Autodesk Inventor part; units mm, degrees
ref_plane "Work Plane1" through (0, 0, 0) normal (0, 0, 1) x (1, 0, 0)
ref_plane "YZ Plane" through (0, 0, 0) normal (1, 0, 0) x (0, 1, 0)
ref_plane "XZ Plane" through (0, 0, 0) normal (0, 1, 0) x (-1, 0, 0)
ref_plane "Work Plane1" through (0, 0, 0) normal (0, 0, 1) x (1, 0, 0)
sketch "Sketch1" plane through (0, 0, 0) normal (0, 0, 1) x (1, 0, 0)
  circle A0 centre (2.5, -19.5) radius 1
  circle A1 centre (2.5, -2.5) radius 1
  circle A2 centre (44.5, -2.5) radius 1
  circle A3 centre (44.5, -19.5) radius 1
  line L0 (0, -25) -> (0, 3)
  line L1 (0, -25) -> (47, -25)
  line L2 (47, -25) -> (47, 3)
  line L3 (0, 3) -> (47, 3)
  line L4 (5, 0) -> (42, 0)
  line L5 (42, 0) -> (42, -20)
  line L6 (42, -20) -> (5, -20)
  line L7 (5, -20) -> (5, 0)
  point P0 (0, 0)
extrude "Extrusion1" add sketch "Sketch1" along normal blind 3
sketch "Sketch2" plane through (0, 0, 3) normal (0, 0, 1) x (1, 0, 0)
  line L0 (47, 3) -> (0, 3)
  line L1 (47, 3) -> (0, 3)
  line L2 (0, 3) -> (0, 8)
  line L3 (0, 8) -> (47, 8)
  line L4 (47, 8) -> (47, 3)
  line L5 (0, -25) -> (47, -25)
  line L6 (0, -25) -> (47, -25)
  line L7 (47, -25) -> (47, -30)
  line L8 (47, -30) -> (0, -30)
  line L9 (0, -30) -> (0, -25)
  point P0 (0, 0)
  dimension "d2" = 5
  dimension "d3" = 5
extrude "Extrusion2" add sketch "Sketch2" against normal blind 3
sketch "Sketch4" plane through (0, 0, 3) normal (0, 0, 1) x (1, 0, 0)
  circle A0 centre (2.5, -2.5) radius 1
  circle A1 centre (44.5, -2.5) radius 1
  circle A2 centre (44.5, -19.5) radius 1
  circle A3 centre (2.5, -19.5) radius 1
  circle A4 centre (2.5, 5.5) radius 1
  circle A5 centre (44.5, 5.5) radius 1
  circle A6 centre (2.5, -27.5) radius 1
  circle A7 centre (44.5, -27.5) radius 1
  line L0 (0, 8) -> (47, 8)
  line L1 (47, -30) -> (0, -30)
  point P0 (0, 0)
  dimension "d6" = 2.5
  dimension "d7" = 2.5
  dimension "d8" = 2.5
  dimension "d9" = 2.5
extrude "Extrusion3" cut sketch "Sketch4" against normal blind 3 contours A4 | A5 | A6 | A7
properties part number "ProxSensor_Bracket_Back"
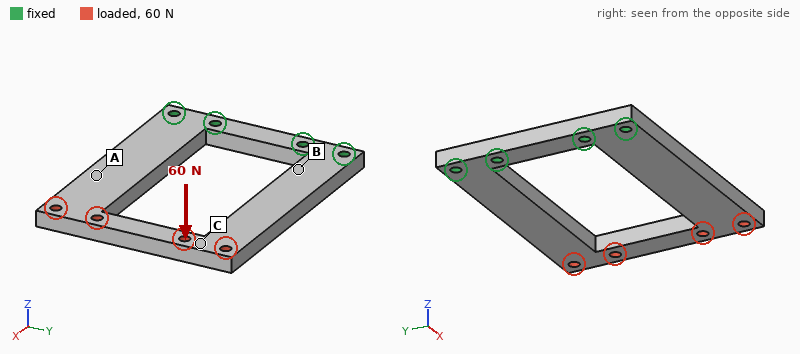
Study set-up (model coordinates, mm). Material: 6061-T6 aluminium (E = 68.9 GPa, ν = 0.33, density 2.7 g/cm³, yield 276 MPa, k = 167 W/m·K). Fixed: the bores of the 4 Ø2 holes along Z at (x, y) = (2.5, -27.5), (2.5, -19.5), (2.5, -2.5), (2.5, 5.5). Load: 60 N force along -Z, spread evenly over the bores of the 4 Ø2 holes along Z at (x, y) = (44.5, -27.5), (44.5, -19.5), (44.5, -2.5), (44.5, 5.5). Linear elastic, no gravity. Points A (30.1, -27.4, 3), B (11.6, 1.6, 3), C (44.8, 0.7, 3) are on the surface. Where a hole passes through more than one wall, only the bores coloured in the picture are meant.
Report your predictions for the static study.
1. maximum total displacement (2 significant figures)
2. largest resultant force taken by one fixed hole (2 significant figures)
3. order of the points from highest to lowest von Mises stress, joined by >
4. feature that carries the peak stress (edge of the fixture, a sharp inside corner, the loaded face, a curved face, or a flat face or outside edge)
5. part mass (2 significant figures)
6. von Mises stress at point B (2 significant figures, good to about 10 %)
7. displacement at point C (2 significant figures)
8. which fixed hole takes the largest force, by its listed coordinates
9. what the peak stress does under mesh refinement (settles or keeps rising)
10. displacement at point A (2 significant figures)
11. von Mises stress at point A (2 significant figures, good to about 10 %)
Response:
0.58 mm
35 N
B > A > C
edge of the fixture
8.3 g
74 MPa
0.54 mm
(2.5, 5.5)
keeps rising
0.26 mm
32 MPa
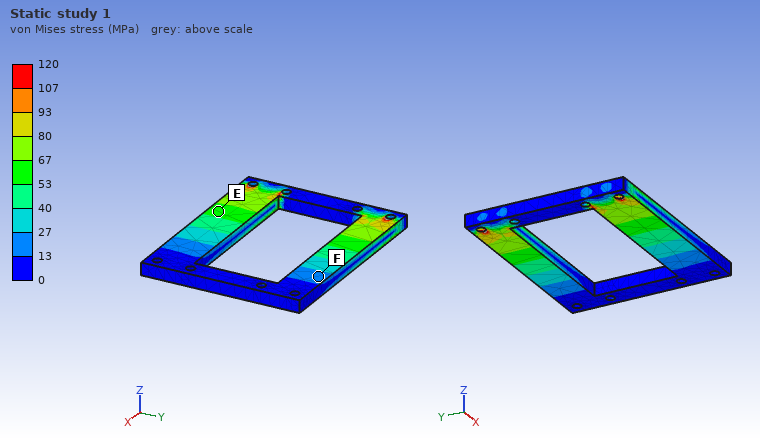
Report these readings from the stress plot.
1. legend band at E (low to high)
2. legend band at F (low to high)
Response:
53 to 67 MPa
13 to 27 MPa
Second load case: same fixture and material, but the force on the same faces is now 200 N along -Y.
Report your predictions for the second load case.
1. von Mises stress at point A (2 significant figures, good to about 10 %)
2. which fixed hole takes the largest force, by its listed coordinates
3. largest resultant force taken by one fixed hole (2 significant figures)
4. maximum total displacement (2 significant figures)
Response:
10.0 MPa
(2.5, -27.5)
480 N
0.11 mm
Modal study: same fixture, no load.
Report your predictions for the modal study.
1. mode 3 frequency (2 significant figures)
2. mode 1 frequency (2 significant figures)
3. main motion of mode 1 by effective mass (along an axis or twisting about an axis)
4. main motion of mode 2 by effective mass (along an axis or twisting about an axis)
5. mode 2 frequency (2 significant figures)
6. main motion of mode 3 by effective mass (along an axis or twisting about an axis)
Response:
4100 Hz
1100 Hz
along Z
twisting about X
2500 Hz
along Y
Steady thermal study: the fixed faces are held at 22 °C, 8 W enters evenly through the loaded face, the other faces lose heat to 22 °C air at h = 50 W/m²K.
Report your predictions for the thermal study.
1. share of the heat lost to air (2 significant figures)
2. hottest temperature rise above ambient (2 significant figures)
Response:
26 %
32 K
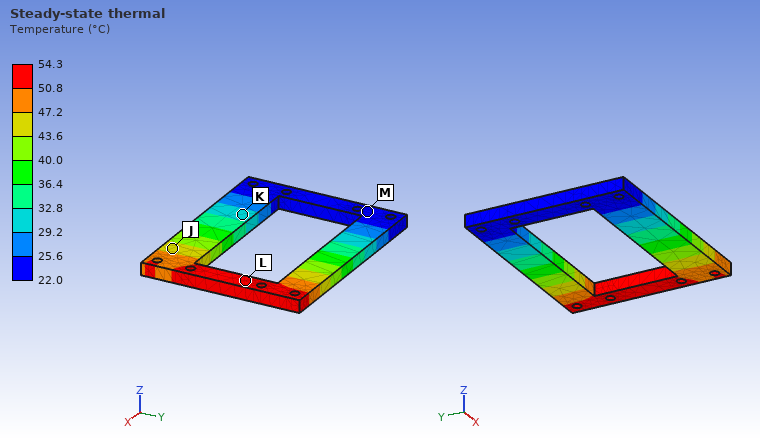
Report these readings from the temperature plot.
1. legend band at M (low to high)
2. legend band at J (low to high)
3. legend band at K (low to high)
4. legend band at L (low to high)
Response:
22.0 to 25.6 °C
43.6 to 47.2 °C
29.2 to 32.8 °C
50.8 to 54.3 °C
